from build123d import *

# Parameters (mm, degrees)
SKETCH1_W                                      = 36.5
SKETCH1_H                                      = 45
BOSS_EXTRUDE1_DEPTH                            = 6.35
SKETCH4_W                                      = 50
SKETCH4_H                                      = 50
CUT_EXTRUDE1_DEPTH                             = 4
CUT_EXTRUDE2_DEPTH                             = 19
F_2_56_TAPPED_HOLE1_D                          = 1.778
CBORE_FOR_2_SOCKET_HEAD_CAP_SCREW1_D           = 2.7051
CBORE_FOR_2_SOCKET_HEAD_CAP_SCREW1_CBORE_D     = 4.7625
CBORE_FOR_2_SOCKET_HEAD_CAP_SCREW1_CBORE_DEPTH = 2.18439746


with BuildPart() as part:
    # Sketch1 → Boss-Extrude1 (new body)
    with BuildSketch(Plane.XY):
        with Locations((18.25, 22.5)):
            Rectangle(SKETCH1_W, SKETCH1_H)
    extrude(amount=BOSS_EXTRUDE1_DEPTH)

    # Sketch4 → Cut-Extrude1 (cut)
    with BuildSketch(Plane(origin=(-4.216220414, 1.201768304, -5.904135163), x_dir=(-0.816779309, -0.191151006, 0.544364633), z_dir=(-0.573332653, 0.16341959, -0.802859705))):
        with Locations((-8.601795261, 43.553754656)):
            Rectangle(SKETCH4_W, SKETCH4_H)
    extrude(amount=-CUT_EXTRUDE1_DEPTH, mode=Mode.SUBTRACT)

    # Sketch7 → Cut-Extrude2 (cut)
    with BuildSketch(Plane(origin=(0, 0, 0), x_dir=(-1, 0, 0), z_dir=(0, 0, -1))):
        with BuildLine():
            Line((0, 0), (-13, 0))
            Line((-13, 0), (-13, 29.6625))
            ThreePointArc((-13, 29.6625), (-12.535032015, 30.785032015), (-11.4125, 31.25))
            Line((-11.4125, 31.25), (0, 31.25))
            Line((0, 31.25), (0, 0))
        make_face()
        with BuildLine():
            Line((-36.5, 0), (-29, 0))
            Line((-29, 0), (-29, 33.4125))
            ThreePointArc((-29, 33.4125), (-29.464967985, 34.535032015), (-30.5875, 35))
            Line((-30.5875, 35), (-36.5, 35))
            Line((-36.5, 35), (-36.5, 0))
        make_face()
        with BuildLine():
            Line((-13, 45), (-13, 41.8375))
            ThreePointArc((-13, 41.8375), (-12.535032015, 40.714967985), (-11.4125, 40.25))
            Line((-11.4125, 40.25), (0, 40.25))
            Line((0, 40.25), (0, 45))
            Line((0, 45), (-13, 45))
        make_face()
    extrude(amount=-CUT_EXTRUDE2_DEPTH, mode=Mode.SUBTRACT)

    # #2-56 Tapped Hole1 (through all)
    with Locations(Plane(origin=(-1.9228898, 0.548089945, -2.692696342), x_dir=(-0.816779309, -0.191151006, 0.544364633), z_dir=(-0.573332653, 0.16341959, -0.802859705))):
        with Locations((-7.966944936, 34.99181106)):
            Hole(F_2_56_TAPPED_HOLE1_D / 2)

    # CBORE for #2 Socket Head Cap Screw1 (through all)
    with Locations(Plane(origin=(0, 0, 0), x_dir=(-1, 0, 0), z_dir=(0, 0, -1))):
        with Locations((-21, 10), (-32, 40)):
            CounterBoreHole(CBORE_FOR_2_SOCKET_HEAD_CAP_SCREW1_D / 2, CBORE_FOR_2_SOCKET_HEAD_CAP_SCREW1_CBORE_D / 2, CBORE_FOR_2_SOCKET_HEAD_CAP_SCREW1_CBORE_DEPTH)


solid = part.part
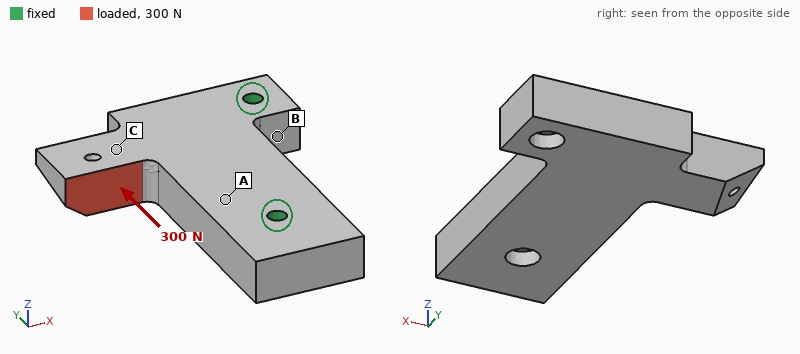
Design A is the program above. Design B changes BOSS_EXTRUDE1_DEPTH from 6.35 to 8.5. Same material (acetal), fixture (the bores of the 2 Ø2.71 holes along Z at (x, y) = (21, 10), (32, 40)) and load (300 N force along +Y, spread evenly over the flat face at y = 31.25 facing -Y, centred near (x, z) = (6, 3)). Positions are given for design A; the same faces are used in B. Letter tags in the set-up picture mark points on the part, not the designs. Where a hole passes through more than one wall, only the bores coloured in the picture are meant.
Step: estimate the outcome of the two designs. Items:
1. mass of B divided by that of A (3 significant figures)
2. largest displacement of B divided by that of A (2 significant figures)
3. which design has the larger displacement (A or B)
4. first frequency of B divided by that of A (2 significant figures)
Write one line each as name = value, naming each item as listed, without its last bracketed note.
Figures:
mass of B divided by that of A = 1.35
largest displacement of B divided by that of A = 0.74
which design has the larger displacement = A
first frequency of B divided by that of A = 1.3
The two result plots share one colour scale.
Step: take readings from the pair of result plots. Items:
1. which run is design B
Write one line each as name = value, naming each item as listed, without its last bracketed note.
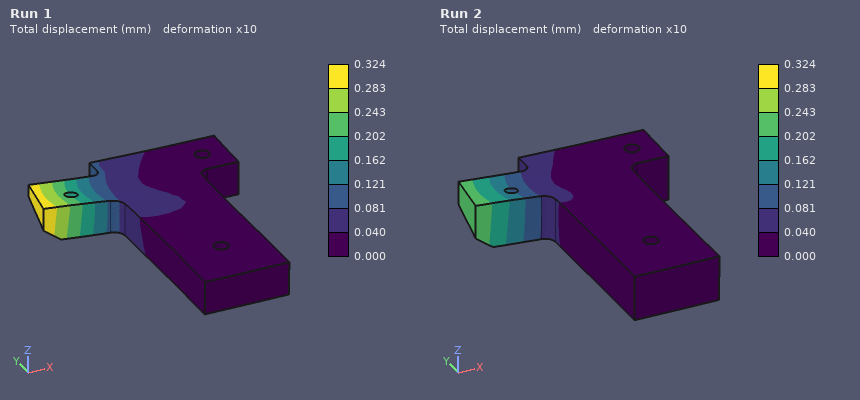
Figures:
which run is design B = Run 2
